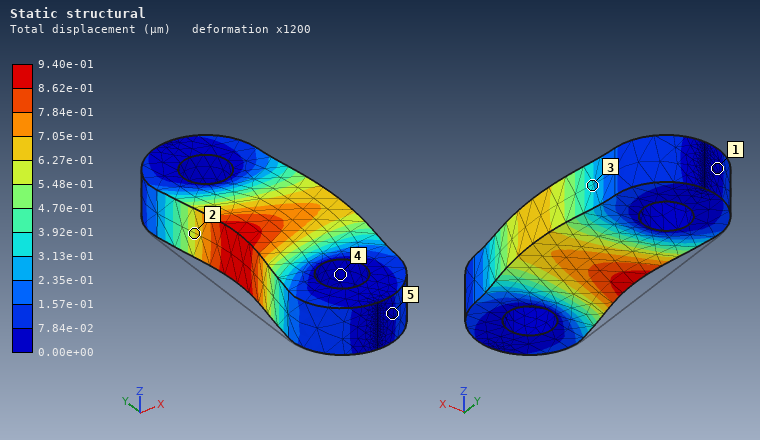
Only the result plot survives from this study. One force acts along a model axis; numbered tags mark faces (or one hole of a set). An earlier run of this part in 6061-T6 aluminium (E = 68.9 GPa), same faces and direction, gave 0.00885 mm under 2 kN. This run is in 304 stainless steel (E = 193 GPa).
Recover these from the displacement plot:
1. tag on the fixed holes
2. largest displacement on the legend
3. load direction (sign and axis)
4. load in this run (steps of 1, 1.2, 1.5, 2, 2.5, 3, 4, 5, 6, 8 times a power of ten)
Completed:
4
9.40e-01 µm
+X
600 N
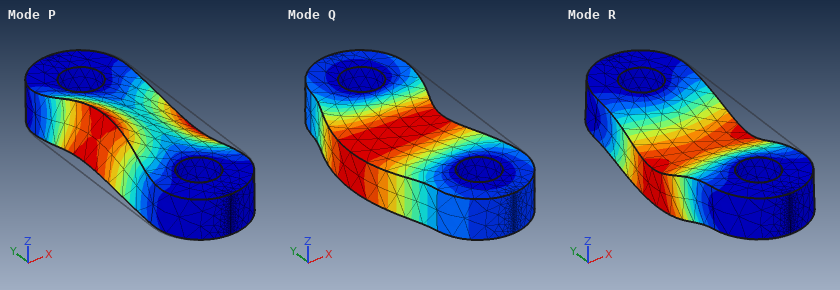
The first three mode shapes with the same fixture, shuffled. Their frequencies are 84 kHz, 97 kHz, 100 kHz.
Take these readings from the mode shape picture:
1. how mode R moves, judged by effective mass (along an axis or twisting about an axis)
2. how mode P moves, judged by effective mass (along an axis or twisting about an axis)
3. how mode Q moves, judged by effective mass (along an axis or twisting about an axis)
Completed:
along Z
twisting about Y
along X
